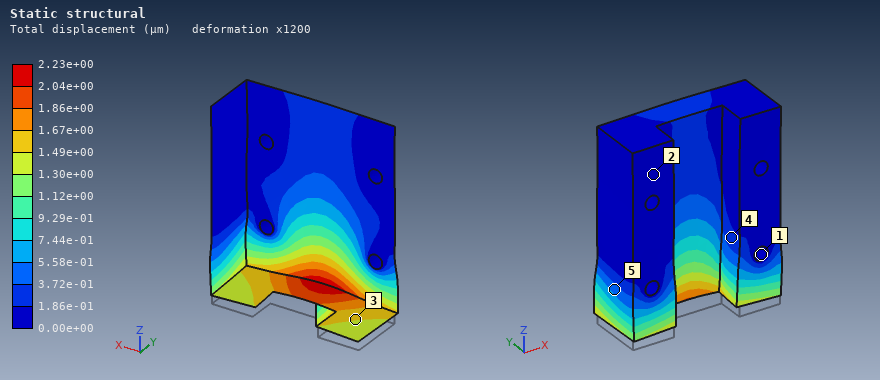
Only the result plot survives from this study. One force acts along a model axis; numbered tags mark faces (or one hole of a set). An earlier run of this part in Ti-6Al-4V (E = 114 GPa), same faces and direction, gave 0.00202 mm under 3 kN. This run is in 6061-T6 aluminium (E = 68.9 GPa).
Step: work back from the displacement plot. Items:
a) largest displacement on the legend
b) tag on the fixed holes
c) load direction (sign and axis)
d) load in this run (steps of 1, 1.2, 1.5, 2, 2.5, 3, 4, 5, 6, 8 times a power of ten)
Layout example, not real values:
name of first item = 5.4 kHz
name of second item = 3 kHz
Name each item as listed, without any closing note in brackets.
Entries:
largest displacement on the legend = 2.23e+00 µm
tag on the fixed holes = 1
load direction = +Z
load in this run = 2 kN
